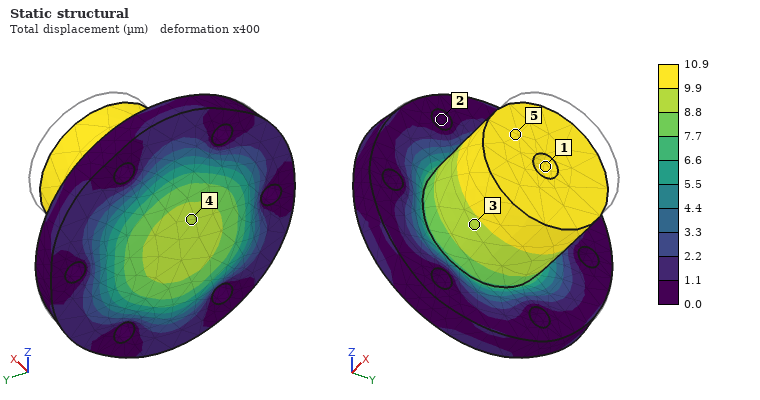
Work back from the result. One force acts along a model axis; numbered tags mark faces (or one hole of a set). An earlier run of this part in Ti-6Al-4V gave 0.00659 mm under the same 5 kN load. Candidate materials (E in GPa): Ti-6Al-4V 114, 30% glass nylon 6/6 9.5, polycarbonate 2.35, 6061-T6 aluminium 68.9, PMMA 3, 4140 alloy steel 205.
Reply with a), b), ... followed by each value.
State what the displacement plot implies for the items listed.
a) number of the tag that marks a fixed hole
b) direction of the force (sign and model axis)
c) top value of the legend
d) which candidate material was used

a) 2
b) -X
c) 10.9 µm
d) 6061-T6 aluminium
